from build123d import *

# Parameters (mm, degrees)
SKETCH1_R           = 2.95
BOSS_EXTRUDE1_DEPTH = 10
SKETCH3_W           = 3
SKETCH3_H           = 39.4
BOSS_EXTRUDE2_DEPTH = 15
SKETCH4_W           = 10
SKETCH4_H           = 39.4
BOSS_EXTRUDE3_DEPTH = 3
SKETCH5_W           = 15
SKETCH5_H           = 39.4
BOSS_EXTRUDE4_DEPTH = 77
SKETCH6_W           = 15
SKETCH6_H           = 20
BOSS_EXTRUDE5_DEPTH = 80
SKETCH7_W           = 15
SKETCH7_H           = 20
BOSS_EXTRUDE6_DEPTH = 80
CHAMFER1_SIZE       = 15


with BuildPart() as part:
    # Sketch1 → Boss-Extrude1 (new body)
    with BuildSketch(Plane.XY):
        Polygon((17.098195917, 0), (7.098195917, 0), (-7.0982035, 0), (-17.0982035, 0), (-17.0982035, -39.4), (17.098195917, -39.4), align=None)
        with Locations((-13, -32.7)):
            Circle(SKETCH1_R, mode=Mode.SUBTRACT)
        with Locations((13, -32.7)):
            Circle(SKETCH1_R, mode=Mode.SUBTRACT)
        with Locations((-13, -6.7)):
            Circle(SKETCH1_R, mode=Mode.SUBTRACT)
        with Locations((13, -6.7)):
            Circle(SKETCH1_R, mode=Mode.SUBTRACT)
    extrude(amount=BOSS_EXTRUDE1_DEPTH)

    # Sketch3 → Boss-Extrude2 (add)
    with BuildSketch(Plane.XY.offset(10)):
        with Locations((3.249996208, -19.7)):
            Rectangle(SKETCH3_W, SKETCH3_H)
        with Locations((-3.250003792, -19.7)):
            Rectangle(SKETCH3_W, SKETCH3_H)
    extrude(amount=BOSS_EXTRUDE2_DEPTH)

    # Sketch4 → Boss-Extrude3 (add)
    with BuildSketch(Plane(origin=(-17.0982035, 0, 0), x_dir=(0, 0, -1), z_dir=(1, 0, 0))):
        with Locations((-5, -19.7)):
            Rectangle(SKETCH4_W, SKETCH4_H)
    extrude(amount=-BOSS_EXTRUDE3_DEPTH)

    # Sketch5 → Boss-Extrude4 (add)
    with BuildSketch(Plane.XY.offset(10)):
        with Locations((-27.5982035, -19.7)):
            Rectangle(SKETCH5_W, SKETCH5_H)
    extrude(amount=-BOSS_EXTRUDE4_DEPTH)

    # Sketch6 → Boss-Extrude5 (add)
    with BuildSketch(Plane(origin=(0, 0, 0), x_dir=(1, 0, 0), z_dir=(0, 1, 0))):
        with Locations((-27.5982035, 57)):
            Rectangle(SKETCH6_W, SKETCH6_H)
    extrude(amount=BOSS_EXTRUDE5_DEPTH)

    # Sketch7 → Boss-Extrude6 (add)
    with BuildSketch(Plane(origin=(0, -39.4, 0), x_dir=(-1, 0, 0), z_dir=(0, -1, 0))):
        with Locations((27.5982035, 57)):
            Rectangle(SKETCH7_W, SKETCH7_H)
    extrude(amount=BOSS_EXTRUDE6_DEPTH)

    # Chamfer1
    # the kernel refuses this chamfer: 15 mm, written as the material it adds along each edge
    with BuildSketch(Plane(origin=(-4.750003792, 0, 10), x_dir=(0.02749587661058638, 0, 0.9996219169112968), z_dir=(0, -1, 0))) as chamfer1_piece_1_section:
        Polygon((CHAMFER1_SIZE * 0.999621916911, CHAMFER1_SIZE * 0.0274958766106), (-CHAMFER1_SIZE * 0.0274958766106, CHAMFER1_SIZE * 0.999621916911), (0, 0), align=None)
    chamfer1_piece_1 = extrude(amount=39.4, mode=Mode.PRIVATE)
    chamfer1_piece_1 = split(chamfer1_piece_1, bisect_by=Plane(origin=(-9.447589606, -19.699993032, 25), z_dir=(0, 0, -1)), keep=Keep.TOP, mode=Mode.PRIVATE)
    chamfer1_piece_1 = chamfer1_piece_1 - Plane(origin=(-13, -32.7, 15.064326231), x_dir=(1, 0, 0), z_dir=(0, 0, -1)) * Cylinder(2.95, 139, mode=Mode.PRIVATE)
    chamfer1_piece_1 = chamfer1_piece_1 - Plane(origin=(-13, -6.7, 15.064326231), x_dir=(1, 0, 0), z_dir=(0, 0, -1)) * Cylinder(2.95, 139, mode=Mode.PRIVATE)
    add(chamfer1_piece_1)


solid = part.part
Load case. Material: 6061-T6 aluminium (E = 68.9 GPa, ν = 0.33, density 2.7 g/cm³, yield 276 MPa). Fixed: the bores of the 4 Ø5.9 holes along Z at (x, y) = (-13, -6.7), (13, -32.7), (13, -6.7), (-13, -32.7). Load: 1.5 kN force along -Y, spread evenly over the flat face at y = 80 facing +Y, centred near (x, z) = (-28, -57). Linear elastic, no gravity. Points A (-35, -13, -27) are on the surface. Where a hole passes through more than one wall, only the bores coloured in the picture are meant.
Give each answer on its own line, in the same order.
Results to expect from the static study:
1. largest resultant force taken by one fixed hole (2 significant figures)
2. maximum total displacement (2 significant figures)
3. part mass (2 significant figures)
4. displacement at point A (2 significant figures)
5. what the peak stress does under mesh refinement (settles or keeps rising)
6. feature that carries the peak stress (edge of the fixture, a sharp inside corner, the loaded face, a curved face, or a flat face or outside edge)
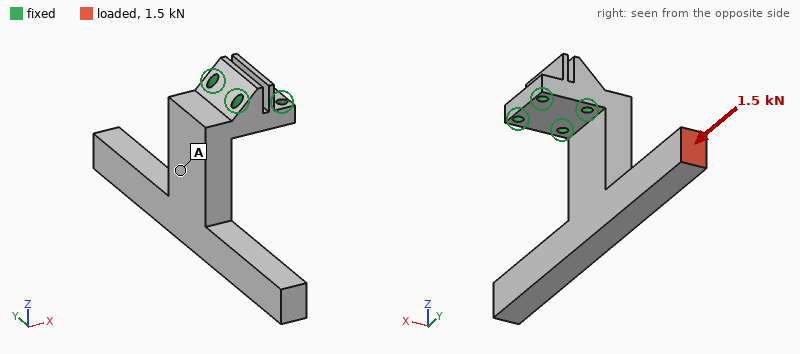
3.2 kN
0.18 mm
310 g
0.033 mm
keeps rising
edge of the fixture
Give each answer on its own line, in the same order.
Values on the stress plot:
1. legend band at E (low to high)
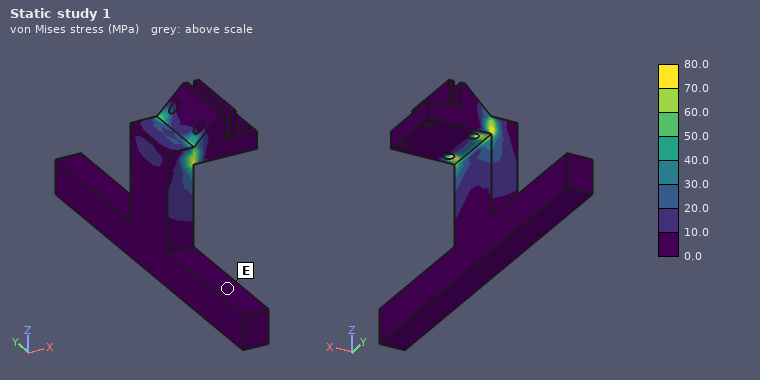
0.0 to 10.0 MPa
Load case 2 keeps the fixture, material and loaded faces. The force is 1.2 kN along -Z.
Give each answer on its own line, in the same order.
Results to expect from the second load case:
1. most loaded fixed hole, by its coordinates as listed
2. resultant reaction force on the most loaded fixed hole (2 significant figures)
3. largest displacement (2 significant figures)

(-13, -6.7)
4.5 kN
0.70 mm
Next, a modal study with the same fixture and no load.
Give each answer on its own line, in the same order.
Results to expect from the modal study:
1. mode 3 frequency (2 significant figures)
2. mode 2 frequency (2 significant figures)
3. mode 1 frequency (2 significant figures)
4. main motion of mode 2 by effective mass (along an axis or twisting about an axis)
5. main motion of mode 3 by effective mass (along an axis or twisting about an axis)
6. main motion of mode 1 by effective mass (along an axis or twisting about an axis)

1100 Hz
750 Hz
700 Hz
twisting about Z
along Y
along X
